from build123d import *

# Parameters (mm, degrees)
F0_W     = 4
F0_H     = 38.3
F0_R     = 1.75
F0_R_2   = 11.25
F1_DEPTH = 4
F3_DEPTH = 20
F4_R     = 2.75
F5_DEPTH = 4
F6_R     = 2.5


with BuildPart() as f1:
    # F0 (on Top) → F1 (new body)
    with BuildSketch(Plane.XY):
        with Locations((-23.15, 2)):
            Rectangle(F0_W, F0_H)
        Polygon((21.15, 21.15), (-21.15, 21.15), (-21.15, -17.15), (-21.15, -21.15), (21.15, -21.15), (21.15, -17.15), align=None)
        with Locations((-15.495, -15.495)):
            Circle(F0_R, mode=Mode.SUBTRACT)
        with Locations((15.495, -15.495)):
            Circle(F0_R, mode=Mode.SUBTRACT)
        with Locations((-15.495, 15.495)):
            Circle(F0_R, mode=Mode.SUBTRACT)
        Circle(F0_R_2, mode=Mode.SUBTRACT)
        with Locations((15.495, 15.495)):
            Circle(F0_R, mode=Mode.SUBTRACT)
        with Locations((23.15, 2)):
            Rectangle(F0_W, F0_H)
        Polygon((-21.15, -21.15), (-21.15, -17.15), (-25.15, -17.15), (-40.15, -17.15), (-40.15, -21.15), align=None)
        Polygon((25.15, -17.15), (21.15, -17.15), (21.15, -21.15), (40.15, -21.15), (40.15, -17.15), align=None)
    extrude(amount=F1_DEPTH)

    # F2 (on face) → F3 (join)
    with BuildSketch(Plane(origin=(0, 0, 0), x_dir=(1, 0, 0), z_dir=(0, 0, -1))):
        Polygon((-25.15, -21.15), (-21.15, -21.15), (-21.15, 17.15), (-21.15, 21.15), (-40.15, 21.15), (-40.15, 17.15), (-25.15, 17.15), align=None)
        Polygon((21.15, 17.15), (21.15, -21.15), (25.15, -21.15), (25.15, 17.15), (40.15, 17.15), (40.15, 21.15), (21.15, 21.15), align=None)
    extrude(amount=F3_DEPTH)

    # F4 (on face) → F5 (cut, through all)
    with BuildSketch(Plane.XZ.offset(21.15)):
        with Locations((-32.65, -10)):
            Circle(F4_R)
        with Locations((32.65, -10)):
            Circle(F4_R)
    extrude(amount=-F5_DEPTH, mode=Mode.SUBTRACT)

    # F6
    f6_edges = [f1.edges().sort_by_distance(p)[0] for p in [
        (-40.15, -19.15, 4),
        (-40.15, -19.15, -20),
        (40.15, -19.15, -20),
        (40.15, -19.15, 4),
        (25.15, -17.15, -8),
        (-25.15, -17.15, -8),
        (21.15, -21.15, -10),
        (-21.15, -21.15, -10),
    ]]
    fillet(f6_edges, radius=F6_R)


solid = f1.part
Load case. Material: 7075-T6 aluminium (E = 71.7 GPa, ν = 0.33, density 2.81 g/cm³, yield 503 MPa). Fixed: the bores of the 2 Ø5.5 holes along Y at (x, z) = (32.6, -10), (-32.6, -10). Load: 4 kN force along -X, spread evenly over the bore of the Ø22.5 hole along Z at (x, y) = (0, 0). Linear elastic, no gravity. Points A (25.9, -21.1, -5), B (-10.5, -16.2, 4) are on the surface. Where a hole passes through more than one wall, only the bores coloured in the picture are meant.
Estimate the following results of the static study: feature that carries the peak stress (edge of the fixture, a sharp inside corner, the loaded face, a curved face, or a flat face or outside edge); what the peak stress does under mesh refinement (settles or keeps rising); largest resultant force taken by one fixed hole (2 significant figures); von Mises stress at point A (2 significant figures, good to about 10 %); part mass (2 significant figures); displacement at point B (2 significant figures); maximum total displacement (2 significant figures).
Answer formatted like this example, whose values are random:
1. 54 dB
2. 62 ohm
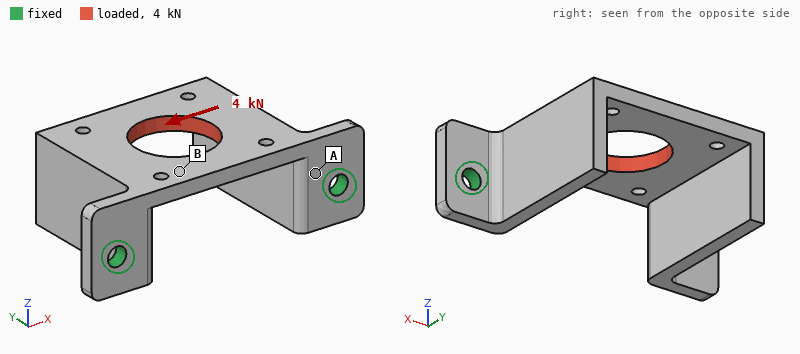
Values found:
1. edge of the fixture
2. keeps rising
3. 2.4 kN
4. 55 MPa
5. 46 g
6. 0.047 mm
7. 0.21 mm
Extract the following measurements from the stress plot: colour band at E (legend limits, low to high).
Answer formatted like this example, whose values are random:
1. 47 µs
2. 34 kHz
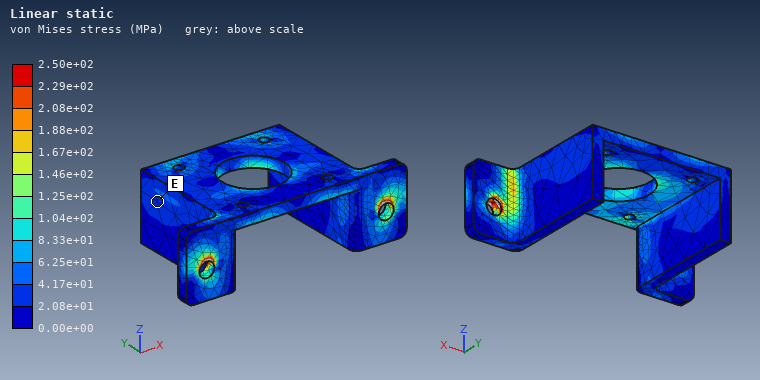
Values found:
1. 2.08e+01 to 4.17e+01 MPa
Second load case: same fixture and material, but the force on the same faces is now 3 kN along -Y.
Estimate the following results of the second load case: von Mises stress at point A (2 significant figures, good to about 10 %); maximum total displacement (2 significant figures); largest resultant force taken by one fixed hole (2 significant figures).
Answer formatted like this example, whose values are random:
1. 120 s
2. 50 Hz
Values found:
1. 66 MPa
2. 0.34 mm
3. 1.6 kN
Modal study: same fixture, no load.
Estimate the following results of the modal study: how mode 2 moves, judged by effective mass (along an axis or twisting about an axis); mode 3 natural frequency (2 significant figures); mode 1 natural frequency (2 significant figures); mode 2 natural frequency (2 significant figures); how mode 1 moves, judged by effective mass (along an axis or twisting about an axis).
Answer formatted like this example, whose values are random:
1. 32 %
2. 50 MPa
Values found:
1. along X
2. 4700 Hz
3. 2100 Hz
4. 2800 Hz
5. along Z
